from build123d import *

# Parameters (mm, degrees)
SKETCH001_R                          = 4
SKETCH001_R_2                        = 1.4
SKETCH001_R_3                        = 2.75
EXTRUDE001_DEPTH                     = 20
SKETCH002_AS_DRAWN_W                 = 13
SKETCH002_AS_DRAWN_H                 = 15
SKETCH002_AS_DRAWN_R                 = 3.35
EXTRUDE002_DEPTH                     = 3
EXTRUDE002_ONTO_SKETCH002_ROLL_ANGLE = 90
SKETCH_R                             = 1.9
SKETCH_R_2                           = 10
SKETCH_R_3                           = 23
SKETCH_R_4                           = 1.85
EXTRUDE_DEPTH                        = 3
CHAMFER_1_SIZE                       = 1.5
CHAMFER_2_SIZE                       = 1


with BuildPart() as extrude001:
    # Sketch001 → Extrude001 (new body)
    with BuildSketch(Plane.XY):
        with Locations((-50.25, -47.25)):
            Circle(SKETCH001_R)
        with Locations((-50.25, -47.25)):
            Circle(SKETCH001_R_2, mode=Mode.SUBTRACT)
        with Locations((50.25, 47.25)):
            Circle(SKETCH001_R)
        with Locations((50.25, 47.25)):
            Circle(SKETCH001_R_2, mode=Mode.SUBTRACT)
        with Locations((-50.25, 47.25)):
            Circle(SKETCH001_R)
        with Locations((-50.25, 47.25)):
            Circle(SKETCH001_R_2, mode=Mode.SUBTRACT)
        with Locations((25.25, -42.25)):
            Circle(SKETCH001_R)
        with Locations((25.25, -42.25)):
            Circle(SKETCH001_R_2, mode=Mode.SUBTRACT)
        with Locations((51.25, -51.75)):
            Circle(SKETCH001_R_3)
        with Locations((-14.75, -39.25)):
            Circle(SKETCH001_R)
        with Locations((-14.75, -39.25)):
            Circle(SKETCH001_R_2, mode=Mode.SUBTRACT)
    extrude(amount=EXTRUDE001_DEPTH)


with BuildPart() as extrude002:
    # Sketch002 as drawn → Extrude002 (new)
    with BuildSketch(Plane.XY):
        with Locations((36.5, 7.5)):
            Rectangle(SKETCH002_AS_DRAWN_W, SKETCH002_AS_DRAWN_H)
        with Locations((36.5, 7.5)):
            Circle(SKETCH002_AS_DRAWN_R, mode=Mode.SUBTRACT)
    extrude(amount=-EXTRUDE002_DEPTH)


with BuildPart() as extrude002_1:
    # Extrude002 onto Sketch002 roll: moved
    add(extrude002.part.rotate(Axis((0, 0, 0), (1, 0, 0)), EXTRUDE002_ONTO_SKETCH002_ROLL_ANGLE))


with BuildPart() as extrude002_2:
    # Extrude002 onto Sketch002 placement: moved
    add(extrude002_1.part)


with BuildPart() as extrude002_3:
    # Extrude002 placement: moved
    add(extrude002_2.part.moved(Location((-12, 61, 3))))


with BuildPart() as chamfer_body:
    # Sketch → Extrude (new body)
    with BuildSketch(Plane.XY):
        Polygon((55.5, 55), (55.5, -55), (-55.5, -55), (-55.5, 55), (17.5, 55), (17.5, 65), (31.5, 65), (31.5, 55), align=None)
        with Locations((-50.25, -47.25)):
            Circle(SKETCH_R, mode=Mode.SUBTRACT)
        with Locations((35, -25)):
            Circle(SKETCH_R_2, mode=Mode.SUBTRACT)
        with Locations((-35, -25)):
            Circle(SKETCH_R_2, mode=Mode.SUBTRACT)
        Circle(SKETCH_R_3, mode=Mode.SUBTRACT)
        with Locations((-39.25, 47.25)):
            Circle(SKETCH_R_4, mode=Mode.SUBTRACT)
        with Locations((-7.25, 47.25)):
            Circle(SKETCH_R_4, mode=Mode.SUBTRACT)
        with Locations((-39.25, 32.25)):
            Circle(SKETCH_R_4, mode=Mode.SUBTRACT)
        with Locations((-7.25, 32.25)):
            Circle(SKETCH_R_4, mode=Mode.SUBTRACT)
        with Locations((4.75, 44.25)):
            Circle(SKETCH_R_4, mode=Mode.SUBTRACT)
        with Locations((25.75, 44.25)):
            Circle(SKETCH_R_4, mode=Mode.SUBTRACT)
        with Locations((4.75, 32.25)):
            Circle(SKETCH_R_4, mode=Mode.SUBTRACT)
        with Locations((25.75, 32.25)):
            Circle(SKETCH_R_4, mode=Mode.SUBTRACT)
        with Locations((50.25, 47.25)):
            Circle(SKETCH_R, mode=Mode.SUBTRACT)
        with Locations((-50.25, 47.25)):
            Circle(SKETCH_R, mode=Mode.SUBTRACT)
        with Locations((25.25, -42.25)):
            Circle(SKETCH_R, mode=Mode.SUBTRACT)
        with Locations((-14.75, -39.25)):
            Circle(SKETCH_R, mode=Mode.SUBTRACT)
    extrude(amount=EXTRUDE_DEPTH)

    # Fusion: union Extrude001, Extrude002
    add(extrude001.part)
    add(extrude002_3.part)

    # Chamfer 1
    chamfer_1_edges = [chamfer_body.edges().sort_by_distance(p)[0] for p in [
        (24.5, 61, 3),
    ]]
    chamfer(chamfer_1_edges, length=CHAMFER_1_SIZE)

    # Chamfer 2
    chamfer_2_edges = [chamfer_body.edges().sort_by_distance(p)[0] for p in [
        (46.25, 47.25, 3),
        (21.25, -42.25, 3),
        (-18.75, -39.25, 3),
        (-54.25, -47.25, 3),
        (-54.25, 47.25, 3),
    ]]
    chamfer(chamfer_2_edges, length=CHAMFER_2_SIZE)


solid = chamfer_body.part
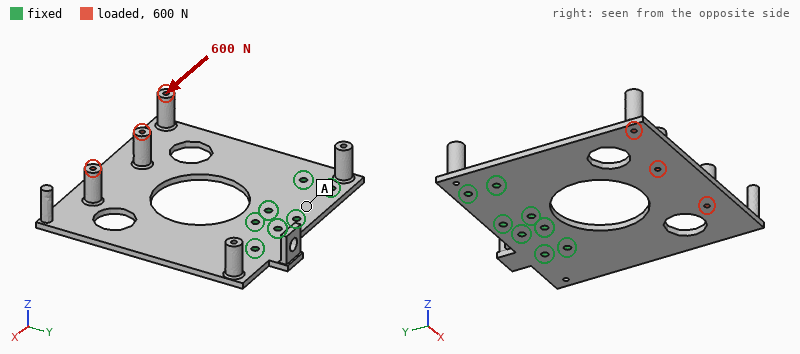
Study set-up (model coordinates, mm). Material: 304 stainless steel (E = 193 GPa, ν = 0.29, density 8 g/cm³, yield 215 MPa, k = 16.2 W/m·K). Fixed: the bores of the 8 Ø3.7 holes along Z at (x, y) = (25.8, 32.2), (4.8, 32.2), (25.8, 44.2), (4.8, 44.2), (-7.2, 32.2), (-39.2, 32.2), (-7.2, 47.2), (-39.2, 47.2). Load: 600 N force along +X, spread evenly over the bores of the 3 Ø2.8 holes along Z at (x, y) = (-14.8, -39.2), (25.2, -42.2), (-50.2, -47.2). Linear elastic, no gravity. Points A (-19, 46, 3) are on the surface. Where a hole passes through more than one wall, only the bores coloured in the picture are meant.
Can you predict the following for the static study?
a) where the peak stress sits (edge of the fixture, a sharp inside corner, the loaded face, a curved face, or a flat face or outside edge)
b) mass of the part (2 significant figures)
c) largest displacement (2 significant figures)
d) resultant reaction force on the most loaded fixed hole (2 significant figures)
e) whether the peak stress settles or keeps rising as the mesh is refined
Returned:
edge of the fixture
280 g
0.29 mm
540 N
keeps rising
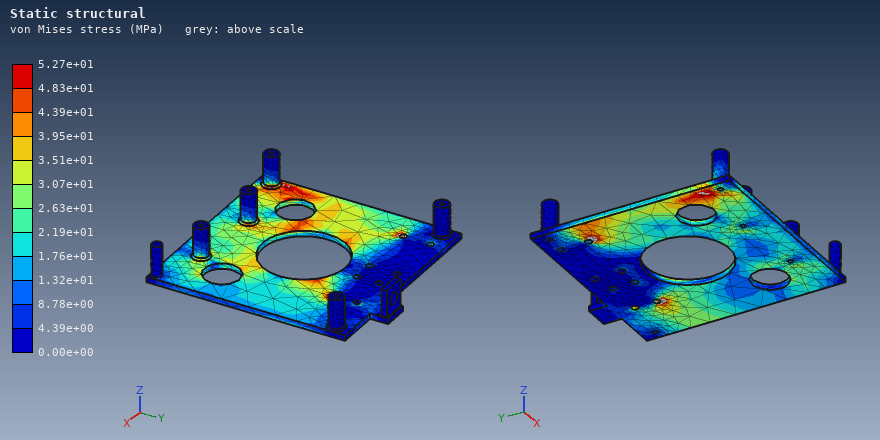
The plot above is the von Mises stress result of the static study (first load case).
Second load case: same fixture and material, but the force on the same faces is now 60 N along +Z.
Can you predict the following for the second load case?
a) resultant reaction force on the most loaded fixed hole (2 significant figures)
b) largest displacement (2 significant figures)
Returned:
92 N
0.38 mm
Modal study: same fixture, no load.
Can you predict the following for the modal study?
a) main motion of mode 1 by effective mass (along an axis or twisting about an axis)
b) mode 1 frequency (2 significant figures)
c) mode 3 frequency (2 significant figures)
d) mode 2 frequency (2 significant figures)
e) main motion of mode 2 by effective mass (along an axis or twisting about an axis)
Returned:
along Z
230 Hz
1200 Hz
480 Hz
twisting about Y
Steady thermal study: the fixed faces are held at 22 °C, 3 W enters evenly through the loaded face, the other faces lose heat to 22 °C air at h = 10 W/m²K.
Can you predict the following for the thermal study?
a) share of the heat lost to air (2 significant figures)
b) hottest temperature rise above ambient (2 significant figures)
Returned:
82 %
40 K
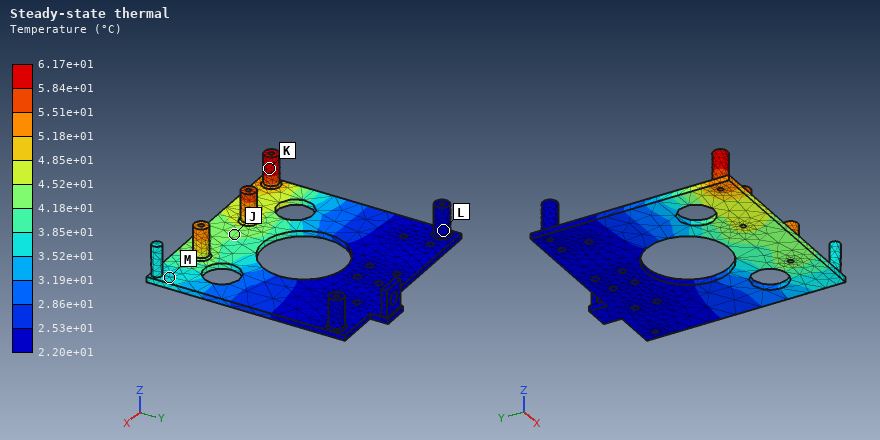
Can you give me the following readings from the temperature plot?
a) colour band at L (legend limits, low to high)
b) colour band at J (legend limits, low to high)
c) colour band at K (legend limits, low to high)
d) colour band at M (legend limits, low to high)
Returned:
2.20e+01 to 2.53e+01 °C
4.18e+01 to 4.52e+01 °C
5.84e+01 to 6.17e+01 °C
3.52e+01 to 3.85e+01 °C
